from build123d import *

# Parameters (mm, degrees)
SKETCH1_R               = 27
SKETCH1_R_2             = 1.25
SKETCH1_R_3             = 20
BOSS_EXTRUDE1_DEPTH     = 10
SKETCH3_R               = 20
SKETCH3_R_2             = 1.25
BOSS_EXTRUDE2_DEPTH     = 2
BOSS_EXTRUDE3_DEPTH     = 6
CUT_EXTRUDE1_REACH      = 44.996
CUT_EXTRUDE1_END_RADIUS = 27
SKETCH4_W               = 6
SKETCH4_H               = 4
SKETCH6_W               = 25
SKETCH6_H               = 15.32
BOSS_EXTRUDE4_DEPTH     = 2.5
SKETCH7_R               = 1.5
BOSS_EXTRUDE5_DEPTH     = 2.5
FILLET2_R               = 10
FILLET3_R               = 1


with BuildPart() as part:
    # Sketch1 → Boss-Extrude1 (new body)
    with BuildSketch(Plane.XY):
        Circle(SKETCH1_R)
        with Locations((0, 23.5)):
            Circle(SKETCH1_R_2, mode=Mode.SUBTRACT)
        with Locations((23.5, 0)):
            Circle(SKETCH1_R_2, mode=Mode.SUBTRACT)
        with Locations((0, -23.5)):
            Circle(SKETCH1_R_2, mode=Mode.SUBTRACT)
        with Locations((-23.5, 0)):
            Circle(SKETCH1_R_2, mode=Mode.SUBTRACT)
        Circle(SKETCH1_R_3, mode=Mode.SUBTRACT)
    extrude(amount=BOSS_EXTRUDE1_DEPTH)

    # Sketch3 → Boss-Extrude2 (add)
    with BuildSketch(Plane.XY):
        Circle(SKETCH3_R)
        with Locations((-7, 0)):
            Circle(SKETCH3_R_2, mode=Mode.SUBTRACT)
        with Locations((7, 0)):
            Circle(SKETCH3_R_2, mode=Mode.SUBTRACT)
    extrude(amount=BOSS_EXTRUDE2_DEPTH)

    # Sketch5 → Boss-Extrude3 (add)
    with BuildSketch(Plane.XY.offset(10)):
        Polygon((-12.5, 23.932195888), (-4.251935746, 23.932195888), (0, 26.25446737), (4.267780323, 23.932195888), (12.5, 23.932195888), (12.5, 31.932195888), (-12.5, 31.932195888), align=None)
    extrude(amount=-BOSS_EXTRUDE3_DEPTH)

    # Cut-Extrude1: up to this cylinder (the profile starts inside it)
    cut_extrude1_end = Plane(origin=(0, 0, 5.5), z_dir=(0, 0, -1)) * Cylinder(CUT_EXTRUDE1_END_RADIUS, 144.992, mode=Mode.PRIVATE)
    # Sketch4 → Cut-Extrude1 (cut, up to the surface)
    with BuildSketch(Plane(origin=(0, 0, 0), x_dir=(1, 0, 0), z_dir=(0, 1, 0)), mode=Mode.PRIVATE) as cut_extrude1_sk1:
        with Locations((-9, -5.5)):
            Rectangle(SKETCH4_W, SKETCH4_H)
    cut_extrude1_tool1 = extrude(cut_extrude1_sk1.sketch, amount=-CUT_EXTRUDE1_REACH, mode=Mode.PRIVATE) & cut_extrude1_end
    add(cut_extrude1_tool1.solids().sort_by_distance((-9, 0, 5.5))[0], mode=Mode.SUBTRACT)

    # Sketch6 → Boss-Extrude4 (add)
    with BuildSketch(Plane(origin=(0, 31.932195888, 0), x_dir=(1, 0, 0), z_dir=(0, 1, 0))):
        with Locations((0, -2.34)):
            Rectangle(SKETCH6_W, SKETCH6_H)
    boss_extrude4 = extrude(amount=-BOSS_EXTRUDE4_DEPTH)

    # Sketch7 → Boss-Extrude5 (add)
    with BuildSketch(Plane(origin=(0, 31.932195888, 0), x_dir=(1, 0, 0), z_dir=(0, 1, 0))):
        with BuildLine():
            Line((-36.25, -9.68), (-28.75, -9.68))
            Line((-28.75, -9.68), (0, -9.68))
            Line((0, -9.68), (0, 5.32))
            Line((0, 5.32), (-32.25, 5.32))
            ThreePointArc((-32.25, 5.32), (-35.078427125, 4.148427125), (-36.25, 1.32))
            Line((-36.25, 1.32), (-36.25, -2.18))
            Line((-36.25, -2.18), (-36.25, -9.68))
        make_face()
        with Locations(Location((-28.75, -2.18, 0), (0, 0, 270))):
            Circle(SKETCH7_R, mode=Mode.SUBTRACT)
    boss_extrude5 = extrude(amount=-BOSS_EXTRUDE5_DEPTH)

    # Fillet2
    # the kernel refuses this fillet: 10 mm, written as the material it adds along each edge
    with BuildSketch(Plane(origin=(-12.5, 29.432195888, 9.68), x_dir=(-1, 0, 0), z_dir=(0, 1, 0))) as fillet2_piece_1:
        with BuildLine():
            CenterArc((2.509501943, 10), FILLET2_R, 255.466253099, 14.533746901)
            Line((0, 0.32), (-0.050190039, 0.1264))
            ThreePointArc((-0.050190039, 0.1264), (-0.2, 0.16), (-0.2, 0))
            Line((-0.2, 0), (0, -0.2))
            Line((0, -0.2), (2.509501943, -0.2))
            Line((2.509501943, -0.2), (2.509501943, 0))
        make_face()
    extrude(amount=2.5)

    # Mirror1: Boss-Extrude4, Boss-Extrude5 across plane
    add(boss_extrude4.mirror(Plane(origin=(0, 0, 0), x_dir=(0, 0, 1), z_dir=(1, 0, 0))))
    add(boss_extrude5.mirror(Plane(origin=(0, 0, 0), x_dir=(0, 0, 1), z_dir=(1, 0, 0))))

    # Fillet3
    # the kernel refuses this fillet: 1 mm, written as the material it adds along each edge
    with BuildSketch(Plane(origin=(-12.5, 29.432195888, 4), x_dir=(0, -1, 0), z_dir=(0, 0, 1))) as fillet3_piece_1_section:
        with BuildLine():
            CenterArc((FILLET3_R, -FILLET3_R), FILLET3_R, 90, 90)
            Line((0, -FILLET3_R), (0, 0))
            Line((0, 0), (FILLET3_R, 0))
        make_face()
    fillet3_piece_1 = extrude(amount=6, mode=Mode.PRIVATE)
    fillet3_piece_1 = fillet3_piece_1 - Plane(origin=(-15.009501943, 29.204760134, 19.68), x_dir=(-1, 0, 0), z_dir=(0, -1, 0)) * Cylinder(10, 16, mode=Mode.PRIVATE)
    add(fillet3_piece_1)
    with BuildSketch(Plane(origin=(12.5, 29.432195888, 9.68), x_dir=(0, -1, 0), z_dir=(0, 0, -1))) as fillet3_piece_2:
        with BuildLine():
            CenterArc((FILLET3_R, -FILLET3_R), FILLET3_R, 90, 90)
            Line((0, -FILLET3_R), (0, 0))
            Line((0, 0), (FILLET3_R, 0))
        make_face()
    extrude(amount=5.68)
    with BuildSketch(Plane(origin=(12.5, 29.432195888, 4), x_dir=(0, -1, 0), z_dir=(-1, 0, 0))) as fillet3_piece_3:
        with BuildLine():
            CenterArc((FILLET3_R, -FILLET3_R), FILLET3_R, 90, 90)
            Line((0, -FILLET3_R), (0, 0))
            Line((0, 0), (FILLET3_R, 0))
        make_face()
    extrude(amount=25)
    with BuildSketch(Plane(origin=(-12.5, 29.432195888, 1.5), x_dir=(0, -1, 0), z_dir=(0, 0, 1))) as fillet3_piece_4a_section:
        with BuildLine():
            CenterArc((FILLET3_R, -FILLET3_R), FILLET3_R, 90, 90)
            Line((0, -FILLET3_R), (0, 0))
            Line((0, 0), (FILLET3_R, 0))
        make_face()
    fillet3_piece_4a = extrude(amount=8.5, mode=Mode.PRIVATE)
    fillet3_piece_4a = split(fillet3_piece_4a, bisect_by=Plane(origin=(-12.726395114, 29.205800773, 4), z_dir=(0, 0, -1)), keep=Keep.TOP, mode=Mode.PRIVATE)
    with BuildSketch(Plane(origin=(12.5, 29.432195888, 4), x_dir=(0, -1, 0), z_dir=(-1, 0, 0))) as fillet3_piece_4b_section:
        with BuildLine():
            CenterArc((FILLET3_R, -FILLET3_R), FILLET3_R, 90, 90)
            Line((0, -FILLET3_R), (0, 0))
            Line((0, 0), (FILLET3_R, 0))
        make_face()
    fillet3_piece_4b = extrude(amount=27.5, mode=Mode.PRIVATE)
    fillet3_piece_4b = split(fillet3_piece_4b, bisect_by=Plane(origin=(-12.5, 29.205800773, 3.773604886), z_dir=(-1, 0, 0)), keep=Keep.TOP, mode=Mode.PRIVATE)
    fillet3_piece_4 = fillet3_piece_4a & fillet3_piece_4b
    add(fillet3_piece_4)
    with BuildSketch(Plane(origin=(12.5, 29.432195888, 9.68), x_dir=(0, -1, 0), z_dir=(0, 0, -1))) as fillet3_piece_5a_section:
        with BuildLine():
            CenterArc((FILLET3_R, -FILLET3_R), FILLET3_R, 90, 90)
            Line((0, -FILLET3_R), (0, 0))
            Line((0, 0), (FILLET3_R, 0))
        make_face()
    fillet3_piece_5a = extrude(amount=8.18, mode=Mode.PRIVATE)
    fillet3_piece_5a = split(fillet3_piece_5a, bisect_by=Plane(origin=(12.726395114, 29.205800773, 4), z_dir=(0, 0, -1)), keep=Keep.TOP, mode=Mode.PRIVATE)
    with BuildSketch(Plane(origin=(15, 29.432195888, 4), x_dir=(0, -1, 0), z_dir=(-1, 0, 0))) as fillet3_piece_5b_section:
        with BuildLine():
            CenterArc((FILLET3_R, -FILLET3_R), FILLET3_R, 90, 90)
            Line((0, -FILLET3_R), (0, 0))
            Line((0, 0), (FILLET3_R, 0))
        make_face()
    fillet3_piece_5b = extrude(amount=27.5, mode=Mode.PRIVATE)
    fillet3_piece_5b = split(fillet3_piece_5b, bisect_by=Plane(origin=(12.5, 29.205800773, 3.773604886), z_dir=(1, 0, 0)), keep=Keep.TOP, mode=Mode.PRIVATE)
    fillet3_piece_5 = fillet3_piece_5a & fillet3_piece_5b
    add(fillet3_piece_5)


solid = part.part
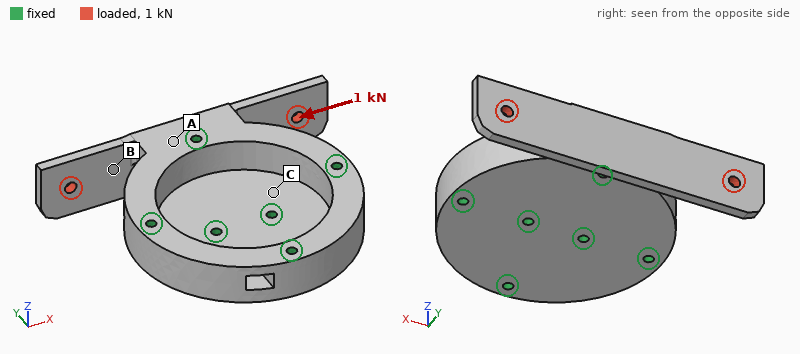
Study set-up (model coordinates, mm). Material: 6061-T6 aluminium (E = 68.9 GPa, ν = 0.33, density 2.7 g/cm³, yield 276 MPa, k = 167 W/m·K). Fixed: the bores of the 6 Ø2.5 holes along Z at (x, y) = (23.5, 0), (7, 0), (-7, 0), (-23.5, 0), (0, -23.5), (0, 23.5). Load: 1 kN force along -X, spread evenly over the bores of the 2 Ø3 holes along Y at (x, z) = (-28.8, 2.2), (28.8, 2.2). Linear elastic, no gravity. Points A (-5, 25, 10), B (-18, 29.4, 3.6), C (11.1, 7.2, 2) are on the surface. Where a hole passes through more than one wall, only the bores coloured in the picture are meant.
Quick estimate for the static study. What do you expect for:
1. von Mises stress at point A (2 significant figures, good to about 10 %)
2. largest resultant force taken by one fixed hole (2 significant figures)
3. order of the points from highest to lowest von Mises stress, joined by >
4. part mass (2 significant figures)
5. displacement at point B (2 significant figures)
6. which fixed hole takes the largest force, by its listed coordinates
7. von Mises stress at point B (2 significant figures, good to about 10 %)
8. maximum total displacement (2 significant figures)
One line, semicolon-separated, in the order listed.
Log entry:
10 MPa; 800 N; B > A > C; 42 g; 16 µm; (0, 23.5); 15 MPa; 35 µm
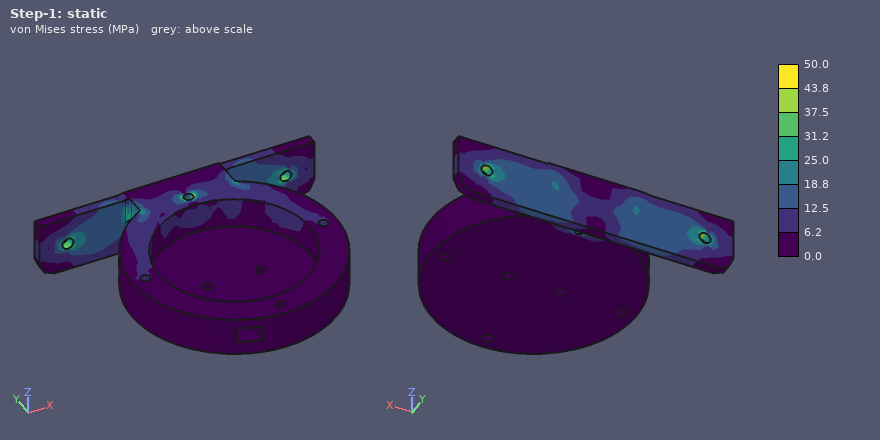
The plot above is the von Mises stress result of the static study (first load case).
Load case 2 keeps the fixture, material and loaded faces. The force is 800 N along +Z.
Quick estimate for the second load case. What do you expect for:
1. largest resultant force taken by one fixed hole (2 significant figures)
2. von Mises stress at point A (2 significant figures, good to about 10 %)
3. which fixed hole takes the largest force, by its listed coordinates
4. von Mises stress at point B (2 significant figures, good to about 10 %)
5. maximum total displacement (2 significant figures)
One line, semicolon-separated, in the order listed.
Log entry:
820 N; 29 MPa; (0, 23.5); 29 MPa; 82 µm
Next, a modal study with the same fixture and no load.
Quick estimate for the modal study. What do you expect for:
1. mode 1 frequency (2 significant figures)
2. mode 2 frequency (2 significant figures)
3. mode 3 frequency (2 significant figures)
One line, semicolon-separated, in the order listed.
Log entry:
3000 Hz; 3000 Hz; 6400 Hz
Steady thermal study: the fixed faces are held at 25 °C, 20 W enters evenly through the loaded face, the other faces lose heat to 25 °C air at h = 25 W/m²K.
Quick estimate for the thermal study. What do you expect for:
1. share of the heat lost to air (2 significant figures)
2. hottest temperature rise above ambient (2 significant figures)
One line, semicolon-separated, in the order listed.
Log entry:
7.8 %; 42 K
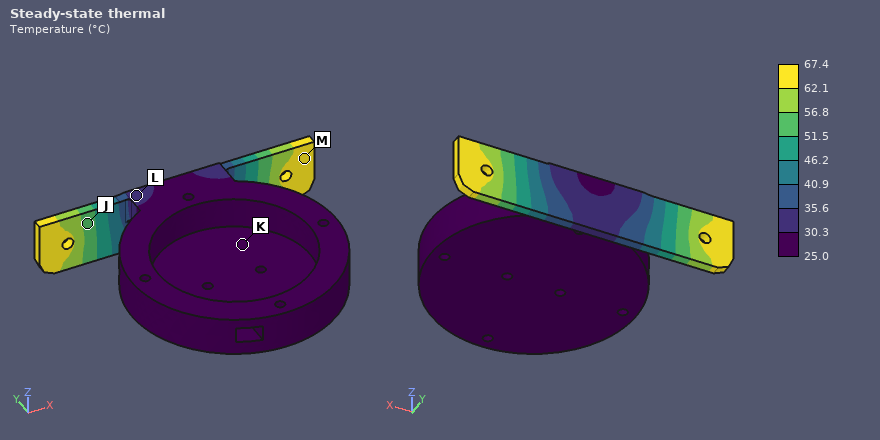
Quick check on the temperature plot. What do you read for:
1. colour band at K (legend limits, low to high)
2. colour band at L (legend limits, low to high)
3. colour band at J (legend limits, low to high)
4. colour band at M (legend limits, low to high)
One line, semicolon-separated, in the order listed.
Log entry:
25.0 to 30.3 °C; 30.3 to 35.6 °C; 51.5 to 56.8 °C; 62.1 to 67.4 °C
